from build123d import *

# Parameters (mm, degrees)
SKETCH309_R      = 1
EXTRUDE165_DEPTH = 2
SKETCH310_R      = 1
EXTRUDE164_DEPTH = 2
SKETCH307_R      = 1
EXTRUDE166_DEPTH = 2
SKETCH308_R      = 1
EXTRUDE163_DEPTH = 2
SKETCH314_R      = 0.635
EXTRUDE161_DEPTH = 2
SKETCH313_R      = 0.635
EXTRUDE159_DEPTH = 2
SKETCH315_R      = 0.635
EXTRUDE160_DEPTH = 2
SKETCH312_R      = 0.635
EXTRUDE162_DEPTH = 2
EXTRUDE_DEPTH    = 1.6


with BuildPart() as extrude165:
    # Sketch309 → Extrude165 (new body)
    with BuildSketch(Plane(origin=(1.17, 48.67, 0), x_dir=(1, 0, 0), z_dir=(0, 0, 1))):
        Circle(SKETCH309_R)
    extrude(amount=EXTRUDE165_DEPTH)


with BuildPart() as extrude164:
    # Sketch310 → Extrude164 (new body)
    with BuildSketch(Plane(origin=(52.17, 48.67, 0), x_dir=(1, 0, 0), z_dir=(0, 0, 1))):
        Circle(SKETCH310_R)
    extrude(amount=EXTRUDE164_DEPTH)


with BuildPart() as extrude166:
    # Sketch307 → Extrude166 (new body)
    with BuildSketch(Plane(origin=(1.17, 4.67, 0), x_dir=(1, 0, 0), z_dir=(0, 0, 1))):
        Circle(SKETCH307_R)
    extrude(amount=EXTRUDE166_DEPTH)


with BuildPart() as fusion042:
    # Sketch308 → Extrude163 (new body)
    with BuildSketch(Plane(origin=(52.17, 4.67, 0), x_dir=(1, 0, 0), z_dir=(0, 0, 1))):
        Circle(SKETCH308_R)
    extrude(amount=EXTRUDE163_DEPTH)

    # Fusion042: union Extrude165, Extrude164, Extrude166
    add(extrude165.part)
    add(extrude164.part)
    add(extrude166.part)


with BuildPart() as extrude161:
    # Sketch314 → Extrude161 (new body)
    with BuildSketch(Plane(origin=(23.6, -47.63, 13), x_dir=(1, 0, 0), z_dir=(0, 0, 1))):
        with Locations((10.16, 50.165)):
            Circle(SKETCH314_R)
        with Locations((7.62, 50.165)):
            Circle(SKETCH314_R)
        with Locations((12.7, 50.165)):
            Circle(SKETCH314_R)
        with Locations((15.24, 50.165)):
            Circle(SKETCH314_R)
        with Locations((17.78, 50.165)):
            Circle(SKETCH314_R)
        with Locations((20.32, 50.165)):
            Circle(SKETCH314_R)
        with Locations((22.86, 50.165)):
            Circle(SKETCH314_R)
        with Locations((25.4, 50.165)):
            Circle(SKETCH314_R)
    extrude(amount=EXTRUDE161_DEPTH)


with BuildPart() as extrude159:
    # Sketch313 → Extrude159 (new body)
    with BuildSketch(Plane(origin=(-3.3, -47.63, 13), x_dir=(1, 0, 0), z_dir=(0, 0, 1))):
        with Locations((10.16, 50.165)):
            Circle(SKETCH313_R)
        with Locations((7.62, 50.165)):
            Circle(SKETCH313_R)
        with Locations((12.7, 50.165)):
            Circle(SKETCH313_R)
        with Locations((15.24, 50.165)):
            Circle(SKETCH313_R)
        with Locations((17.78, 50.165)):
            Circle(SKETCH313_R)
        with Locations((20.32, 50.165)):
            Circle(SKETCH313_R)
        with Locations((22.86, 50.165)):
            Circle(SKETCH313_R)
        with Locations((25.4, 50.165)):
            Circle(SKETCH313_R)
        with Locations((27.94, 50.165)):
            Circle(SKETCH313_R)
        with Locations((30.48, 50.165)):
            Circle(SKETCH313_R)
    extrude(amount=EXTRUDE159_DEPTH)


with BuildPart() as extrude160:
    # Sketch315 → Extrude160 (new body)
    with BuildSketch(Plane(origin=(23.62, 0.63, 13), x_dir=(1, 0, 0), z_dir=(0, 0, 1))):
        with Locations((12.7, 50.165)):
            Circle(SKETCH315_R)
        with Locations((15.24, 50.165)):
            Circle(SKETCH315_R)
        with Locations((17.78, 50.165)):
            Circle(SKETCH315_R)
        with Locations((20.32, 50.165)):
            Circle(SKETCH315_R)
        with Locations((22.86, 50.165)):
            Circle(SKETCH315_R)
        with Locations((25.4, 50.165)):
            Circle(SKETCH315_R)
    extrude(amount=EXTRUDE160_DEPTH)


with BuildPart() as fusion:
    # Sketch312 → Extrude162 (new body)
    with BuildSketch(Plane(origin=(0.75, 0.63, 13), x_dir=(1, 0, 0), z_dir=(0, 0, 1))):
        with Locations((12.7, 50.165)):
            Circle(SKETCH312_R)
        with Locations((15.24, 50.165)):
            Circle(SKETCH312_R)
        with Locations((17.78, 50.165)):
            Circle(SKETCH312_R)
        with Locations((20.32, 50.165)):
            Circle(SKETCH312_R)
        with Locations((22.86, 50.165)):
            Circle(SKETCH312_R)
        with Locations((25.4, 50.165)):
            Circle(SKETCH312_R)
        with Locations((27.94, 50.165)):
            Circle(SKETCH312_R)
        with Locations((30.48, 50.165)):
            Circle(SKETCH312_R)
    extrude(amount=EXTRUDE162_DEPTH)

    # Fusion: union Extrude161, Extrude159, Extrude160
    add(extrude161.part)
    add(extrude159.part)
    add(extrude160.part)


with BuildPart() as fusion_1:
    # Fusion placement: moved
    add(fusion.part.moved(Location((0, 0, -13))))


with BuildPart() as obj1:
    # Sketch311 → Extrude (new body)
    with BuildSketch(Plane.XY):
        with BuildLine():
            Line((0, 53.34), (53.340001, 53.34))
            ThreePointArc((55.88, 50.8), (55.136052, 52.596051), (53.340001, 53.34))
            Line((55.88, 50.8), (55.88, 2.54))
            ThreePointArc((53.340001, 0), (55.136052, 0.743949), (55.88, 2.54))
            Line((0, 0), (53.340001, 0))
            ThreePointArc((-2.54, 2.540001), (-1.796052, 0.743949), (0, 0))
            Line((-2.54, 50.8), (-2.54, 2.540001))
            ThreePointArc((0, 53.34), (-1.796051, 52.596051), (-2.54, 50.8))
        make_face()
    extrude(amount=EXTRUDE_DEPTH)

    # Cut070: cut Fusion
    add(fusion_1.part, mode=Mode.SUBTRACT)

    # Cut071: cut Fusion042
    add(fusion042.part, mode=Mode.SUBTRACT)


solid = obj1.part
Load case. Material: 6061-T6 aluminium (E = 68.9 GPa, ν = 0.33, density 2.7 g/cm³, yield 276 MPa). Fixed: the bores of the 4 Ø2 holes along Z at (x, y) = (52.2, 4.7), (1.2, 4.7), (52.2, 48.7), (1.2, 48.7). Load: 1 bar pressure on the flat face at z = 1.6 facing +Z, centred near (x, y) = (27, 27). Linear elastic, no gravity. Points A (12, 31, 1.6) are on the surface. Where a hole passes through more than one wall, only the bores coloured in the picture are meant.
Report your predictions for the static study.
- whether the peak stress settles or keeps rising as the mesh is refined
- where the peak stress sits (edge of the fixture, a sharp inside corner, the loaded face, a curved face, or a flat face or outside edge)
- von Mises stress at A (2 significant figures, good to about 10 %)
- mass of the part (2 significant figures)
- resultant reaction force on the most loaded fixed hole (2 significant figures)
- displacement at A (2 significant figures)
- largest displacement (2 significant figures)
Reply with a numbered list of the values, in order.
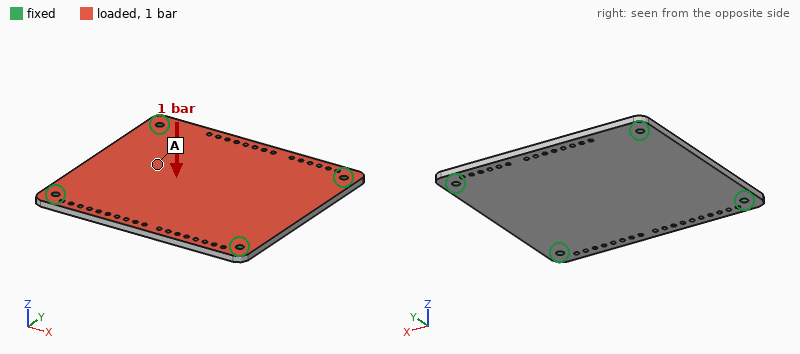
1. keeps rising
2. edge of the fixture
3. 22 MPa
4. 13 g
5. 77 N
6. 0.12 mm
7. 0.16 mm
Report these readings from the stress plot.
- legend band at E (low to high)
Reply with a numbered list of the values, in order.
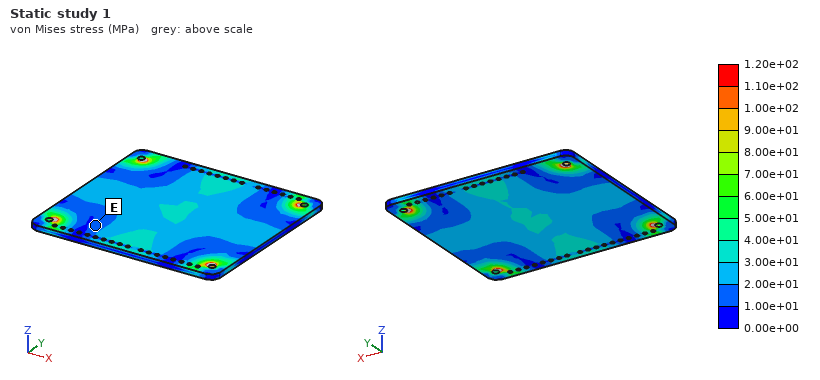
1. 1.00e+01 to 2.00e+01 MPa
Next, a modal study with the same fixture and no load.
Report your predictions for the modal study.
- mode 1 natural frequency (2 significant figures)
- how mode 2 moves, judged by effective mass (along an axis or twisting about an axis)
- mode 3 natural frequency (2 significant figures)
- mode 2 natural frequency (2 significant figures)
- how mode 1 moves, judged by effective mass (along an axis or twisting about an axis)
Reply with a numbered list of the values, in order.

1. 2300 Hz
2. twisting about X
3. 4400 Hz
4. 3600 Hz
5. along Z
